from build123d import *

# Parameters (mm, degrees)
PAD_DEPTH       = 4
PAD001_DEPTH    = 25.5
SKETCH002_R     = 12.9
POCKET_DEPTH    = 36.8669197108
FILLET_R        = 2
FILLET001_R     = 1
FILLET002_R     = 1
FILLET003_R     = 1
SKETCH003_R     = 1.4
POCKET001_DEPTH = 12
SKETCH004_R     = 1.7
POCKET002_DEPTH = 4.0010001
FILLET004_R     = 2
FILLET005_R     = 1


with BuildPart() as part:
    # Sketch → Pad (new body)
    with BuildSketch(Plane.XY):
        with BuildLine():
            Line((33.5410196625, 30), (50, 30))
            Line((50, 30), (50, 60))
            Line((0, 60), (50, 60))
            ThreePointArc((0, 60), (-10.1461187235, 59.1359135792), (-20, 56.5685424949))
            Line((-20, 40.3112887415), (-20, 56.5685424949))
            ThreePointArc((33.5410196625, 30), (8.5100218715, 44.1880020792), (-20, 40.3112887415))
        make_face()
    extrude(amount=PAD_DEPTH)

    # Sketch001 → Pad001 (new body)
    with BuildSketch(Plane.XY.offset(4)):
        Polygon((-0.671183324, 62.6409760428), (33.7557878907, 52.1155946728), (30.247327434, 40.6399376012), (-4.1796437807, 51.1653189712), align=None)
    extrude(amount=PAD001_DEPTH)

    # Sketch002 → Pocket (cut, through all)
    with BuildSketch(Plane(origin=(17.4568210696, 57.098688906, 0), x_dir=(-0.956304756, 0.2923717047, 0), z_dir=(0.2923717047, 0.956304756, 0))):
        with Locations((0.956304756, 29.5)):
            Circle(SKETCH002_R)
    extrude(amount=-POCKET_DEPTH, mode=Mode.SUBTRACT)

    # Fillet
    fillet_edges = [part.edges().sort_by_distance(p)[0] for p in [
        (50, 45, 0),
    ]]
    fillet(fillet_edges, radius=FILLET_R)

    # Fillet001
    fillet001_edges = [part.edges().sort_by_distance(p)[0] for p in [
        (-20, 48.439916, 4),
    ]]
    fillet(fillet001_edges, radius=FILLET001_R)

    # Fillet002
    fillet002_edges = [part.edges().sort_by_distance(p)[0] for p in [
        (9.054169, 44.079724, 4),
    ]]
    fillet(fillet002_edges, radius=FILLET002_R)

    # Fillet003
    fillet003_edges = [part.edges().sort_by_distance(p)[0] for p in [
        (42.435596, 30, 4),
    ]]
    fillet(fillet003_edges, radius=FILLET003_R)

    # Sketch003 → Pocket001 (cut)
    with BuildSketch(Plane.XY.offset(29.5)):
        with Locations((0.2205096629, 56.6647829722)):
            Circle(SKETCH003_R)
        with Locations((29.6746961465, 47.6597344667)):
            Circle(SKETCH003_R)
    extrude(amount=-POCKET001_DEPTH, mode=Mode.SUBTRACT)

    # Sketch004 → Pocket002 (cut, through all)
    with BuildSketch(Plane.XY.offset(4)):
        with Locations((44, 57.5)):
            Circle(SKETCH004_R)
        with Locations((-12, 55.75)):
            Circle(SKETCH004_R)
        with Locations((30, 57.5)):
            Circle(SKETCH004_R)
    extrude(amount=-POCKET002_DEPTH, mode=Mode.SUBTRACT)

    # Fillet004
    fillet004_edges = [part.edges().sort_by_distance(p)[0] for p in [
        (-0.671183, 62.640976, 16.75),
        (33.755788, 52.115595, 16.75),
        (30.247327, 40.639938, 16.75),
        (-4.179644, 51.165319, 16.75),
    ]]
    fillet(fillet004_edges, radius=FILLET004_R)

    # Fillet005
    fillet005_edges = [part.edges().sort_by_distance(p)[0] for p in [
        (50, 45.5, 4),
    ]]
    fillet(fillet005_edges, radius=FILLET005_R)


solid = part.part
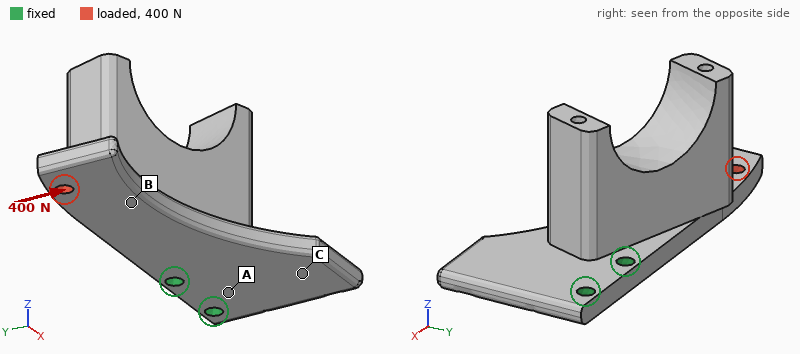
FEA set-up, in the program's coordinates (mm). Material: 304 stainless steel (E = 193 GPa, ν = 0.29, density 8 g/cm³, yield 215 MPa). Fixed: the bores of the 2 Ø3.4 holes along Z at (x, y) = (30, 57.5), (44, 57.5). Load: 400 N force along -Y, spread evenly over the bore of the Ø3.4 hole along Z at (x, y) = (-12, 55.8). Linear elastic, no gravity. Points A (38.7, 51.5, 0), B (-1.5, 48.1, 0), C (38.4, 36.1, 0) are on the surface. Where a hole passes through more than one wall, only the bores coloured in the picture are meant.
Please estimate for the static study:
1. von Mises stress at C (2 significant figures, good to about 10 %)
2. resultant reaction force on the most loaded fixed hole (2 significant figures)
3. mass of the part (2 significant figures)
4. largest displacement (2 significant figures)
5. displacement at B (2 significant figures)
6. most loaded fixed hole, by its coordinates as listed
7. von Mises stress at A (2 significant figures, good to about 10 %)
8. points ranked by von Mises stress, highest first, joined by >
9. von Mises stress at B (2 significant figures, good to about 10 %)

7.0 MPa
1.4 kN
110 g
41 µm
21 µm
(30, 57.5)
28 MPa
A > B > C
16 MPa
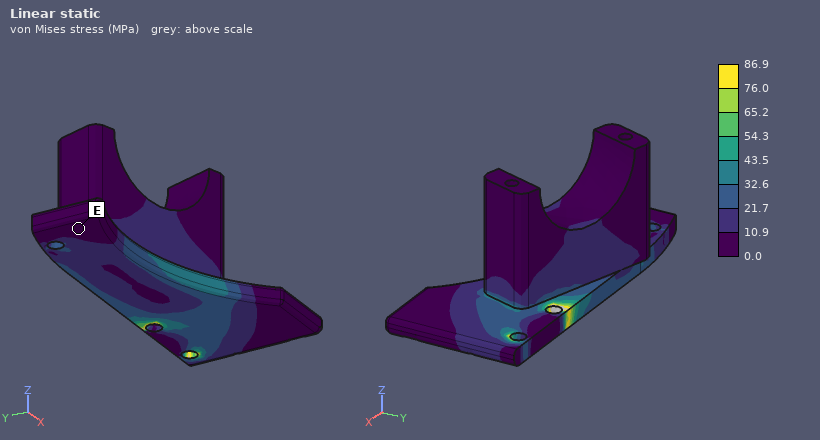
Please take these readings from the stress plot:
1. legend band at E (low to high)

0.0 to 10.9 MPa
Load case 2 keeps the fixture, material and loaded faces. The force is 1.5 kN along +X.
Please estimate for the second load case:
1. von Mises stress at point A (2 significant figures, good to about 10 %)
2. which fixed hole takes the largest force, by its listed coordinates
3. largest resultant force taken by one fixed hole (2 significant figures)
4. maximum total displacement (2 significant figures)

7.8 MPa
(30, 57.5)
1.3 kN
19 µm
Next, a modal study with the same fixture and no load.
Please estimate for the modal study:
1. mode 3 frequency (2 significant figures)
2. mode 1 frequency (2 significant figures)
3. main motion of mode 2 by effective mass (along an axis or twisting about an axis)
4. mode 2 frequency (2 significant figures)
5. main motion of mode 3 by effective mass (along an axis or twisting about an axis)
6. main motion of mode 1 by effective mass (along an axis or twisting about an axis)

4400 Hz
1600 Hz
along Y
2500 Hz
along Y
along Z
